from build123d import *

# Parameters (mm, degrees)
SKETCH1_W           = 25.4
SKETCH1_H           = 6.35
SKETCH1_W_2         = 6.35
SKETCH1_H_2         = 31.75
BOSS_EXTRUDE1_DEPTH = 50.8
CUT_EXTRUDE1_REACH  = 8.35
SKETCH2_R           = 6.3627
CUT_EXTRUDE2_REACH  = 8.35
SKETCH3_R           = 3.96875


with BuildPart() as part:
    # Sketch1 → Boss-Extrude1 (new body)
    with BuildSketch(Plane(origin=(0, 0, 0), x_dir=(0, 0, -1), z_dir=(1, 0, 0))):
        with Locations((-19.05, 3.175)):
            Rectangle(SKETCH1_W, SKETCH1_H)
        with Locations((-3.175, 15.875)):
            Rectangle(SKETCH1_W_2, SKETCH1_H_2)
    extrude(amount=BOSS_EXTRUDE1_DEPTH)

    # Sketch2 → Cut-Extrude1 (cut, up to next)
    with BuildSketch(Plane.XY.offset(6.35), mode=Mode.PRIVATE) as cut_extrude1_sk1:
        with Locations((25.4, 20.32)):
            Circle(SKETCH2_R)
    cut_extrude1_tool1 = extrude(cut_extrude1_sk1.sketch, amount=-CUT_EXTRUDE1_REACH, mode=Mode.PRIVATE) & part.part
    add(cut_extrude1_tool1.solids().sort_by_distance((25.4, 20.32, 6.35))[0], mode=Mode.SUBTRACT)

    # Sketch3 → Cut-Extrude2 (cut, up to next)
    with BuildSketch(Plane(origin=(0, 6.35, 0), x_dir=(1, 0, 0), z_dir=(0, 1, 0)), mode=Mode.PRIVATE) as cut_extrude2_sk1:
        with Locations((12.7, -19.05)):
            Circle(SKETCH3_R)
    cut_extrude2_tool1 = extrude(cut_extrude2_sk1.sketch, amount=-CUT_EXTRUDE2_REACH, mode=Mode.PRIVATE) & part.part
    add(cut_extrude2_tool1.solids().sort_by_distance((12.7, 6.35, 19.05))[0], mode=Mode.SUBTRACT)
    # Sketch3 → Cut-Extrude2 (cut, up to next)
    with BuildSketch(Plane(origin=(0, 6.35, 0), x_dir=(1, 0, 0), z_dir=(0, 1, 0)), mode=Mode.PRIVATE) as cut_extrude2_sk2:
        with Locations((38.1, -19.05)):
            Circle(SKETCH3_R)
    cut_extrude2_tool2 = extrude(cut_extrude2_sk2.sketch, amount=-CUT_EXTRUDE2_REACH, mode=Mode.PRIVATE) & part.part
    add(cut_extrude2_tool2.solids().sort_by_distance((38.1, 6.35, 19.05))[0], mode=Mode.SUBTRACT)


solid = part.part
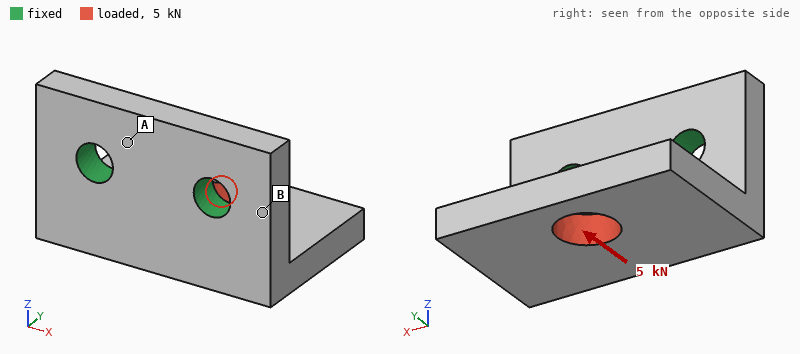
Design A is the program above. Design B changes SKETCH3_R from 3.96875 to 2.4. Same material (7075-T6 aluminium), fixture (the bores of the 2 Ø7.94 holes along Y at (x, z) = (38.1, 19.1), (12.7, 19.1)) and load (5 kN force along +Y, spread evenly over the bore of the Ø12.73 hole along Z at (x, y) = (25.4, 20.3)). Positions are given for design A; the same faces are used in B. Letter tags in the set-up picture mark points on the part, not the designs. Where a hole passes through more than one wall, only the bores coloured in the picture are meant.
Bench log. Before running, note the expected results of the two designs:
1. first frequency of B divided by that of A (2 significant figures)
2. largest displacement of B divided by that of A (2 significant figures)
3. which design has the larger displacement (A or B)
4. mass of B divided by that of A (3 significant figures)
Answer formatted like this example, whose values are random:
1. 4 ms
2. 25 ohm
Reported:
1. 0.91
2. 1.4
3. B
4. 1.02
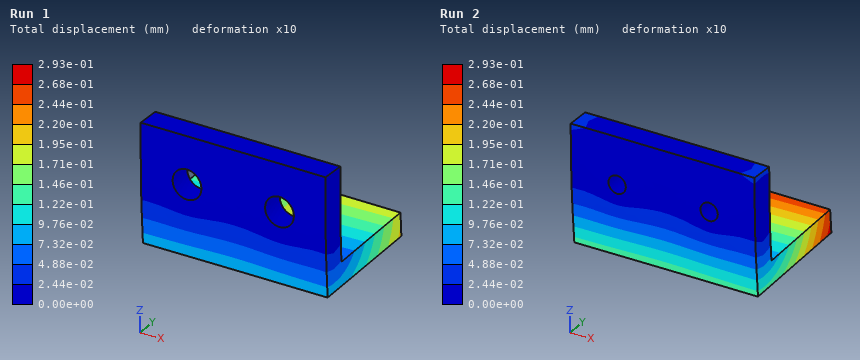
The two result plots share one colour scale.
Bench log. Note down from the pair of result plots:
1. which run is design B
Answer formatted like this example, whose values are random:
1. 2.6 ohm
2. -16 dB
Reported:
1. Run 2
